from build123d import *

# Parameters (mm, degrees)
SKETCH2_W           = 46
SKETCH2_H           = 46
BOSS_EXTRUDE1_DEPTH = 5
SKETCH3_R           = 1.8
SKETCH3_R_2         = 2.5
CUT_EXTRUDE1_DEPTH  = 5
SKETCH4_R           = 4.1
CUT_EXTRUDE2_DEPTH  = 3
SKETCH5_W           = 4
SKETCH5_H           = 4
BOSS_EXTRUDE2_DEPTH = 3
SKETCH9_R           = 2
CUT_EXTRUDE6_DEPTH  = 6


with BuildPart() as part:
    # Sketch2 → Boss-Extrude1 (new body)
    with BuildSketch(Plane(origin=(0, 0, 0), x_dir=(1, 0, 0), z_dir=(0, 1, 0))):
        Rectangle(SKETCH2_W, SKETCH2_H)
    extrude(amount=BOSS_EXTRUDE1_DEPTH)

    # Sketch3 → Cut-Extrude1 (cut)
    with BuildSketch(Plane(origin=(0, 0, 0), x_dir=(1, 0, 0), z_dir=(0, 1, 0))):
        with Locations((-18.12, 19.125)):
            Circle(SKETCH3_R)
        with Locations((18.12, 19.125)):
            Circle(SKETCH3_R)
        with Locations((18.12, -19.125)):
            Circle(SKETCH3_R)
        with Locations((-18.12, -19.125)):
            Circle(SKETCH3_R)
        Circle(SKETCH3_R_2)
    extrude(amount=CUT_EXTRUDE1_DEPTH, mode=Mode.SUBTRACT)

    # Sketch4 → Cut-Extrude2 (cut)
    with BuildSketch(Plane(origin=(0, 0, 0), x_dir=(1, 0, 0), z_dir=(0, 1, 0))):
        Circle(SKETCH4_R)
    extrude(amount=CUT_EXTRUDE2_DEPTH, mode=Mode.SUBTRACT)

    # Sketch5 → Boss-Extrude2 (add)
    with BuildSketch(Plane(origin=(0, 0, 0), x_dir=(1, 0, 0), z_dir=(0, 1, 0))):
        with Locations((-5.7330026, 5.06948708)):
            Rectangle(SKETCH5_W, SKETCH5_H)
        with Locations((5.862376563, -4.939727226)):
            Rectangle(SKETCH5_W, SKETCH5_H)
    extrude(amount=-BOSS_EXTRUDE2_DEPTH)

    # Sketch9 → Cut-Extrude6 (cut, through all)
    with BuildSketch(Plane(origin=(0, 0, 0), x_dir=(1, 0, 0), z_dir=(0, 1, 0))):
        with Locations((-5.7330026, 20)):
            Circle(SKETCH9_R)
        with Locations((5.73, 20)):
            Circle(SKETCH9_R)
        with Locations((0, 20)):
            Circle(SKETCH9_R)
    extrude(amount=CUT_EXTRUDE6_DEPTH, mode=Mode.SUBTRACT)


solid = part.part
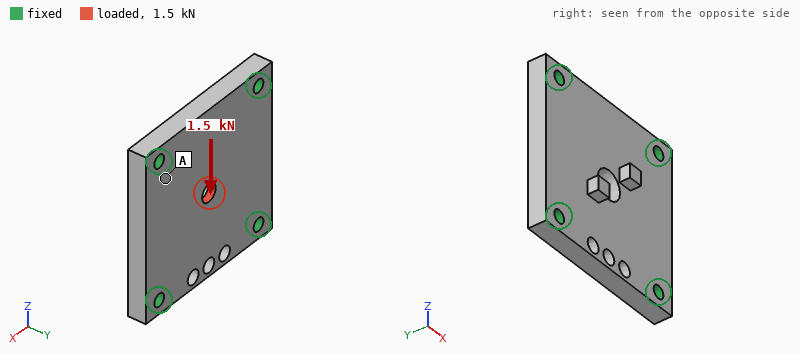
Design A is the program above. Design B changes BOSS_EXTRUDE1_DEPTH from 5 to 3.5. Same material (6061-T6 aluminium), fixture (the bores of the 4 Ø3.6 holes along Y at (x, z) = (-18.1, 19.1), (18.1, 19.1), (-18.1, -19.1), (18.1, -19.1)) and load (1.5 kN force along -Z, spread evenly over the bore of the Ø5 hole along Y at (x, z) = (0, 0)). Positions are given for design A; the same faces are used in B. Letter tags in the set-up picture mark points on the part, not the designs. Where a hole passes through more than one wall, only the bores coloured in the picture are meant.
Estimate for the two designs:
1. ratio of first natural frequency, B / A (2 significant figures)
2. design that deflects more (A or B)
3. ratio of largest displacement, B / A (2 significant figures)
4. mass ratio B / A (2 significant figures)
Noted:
0.75
B
2.4
0.70
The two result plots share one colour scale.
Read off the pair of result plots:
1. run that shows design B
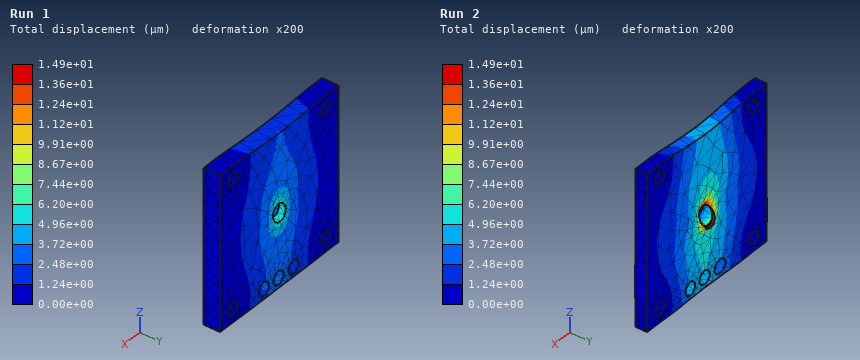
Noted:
Run 2
